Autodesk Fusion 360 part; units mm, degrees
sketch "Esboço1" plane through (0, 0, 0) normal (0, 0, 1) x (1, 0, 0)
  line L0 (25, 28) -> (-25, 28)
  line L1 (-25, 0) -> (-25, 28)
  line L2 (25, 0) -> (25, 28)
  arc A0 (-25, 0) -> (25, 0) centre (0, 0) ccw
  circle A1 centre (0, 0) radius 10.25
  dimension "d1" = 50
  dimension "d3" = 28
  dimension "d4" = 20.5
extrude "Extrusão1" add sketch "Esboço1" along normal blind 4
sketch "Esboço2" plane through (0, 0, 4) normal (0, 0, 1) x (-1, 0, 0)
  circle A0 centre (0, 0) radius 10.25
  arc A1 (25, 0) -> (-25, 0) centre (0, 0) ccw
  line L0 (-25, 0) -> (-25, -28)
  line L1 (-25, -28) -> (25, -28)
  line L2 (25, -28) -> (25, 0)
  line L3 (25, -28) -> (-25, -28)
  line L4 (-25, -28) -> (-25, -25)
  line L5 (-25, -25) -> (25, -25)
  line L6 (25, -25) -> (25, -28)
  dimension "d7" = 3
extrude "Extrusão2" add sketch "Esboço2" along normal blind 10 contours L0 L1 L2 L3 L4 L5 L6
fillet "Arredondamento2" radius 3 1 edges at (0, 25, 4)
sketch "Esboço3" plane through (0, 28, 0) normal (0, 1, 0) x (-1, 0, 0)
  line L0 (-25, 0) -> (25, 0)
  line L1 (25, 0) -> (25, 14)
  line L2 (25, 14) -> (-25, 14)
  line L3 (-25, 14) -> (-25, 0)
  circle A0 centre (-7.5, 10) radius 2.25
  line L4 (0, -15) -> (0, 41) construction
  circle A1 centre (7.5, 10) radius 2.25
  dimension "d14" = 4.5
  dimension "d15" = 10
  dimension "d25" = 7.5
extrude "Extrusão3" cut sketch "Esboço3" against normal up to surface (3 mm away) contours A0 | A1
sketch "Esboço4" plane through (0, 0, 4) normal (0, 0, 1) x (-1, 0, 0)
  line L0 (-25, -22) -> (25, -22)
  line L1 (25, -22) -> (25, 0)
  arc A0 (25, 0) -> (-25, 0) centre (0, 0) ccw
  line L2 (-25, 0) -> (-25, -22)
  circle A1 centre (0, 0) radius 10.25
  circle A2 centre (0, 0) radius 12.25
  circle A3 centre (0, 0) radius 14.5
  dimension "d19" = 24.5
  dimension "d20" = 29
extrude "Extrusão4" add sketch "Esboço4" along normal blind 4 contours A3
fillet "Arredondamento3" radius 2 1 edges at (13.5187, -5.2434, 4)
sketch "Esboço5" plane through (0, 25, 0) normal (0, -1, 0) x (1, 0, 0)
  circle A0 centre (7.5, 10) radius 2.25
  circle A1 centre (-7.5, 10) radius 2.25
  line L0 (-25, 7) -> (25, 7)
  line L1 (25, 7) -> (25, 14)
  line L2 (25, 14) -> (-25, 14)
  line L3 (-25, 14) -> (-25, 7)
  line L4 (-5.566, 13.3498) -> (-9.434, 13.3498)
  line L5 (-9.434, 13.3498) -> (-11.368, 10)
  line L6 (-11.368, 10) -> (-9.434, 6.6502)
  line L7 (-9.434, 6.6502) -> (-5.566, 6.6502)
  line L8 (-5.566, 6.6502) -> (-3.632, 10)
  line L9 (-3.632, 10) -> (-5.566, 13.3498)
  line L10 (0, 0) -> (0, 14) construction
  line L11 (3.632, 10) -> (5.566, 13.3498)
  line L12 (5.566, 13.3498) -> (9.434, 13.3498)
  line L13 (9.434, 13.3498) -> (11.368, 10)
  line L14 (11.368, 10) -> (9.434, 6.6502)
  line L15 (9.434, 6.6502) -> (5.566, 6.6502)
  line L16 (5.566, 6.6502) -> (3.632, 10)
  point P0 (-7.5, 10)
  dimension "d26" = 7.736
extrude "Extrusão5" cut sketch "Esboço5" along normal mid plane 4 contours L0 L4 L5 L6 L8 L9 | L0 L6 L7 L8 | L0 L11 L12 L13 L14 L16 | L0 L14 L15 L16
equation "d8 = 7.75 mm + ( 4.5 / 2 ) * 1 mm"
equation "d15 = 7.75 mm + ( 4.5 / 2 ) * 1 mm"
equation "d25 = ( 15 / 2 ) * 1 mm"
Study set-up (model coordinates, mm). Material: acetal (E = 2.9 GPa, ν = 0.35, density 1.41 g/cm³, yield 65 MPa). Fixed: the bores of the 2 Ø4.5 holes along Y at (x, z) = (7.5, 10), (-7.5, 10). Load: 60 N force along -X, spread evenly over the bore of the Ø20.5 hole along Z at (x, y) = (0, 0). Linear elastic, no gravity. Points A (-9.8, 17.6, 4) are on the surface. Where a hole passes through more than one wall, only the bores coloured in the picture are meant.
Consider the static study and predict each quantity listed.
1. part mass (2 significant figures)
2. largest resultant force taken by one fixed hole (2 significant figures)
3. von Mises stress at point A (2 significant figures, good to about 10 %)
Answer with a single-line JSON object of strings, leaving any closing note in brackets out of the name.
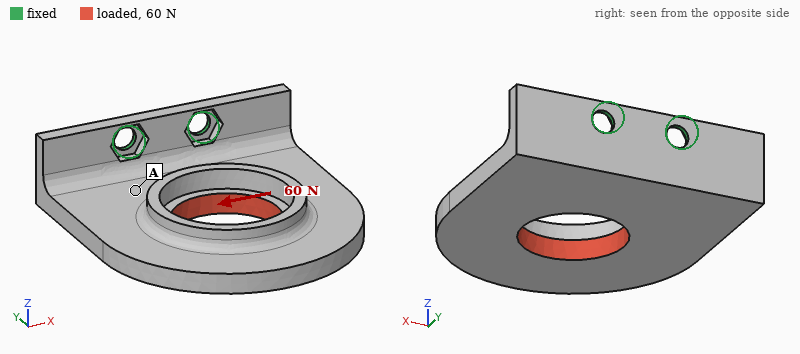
{"part mass": "15 g", "largest resultant force taken by one fixed hole": "110 N", "von Mises stress at point A": "3.5 MPa"}
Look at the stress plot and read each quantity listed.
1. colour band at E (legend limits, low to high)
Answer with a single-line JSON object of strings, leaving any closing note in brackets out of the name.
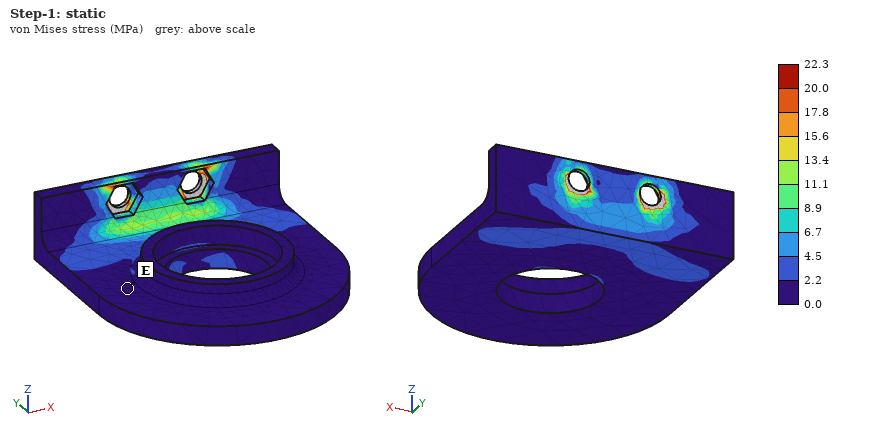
{"colour band at E": "0.0 to 2.2 MPa"}
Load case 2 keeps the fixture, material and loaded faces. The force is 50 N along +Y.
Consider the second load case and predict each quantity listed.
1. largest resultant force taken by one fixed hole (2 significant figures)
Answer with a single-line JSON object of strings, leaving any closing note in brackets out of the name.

{"largest resultant force taken by one fixed hole": "25 N"}
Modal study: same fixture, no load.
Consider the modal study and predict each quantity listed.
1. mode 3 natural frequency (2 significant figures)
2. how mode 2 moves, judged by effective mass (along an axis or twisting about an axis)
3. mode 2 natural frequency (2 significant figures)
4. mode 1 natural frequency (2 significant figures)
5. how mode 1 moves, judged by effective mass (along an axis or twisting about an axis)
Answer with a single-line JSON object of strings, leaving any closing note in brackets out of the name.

{"mode 3 natural frequency": "990 Hz", "how mode 2 moves, judged by effective mass": "along X", "mode 2 natural frequency": "530 Hz", "mode 1 natural frequency": "200 Hz", "how mode 1 moves, judged by effective mass": "along Z"}
